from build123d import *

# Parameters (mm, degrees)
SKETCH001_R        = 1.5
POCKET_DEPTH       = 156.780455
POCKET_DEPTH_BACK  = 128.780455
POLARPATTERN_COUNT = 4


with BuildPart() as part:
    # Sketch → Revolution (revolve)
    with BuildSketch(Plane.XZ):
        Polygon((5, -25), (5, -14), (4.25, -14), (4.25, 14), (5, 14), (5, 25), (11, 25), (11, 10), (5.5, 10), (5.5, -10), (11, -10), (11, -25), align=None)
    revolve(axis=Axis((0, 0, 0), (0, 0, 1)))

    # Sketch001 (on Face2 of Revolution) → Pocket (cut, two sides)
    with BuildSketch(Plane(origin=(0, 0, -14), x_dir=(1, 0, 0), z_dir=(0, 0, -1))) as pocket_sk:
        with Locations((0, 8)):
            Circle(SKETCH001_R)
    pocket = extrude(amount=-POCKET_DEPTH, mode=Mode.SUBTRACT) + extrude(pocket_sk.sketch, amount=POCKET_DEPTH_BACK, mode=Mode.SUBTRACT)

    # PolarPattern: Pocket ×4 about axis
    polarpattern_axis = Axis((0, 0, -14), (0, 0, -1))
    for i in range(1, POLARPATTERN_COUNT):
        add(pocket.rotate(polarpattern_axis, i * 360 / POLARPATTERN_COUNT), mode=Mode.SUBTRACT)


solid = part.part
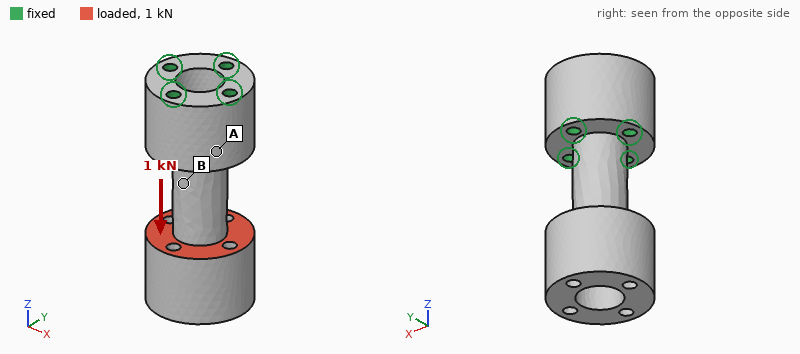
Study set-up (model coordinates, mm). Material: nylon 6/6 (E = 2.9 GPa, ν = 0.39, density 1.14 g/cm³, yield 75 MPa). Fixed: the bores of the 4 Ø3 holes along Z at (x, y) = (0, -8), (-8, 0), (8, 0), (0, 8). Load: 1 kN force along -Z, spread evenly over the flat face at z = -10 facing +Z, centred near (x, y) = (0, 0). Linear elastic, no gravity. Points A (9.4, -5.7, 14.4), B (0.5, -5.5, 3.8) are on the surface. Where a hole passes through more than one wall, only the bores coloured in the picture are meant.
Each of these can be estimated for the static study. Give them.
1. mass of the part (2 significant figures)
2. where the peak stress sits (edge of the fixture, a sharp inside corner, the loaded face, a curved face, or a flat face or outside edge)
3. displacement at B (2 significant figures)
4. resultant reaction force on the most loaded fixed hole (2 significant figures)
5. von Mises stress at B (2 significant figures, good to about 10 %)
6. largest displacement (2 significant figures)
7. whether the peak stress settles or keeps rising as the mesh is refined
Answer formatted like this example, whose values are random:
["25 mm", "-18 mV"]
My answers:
["10 g", "edge of the fixture", "0.076 mm", "270 N", "26 MPa", "0.23 mm", "keeps rising"]
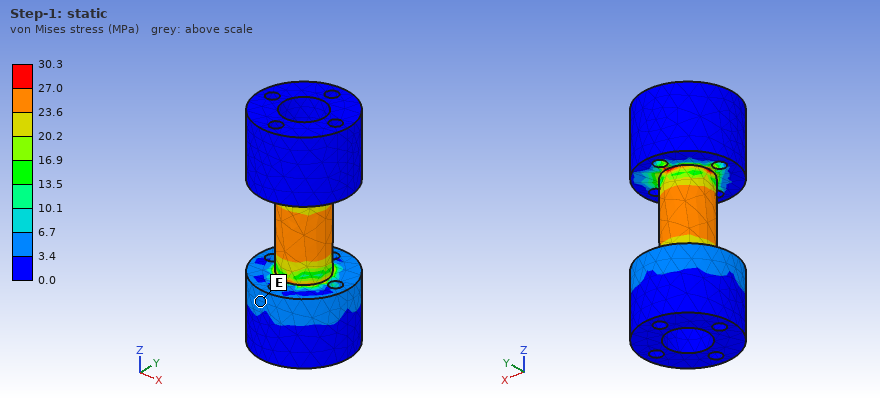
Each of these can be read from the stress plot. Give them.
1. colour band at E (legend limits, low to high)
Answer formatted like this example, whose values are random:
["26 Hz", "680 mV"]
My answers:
["3.4 to 6.7 MPa"]
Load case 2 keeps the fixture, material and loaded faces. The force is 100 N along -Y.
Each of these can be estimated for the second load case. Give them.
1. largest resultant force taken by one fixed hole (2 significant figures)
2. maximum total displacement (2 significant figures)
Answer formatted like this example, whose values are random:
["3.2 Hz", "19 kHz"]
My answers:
["160 N", "0.63 mm"]
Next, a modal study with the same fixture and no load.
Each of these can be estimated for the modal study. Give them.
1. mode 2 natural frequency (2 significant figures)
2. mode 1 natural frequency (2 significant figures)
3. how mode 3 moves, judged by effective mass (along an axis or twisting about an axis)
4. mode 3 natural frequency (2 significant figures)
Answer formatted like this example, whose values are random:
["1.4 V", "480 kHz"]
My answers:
["820 Hz", "820 Hz", "twisting about Z", "1800 Hz"]
